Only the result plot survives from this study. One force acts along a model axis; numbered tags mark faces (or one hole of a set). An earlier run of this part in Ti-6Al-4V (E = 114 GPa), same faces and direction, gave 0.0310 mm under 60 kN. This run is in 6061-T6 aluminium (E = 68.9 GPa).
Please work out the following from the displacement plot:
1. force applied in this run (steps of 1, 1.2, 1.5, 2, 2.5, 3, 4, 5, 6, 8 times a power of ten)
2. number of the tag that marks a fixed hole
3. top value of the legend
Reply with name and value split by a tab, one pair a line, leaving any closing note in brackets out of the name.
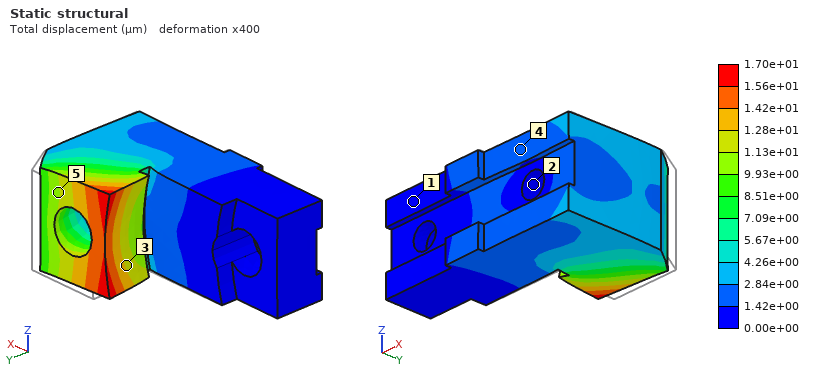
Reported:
force applied in this run	20 kN
number of the tag that marks a fixed hole	2
top value of the legend	1.70e+01 µm
